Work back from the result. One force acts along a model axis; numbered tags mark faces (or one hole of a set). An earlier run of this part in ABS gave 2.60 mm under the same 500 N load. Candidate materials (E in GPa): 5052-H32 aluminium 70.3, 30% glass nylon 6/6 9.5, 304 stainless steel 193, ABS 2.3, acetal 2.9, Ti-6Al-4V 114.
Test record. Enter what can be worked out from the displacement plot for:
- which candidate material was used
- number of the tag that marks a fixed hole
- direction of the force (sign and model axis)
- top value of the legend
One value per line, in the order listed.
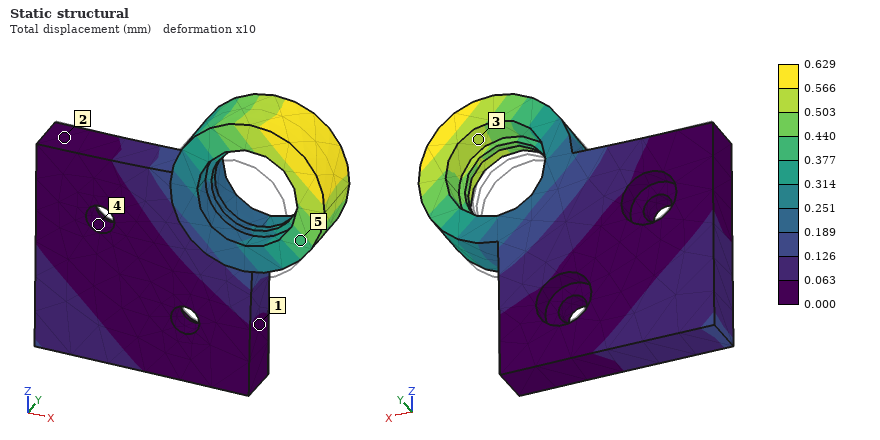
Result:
30% glass nylon 6/6
4
+Y
0.629 mm
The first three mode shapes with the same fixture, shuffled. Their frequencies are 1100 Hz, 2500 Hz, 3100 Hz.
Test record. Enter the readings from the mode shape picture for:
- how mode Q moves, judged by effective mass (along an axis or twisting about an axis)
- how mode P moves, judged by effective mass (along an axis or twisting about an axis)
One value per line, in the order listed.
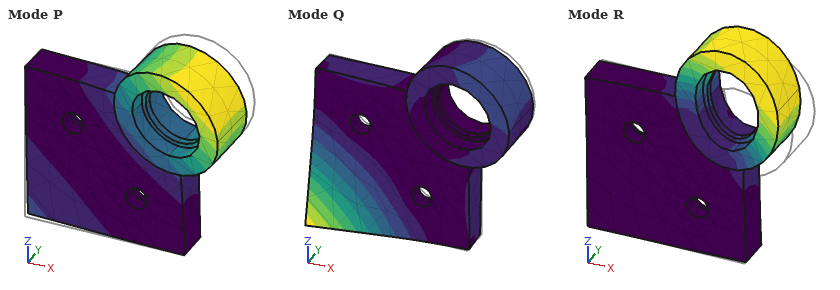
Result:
along Y
along Y
